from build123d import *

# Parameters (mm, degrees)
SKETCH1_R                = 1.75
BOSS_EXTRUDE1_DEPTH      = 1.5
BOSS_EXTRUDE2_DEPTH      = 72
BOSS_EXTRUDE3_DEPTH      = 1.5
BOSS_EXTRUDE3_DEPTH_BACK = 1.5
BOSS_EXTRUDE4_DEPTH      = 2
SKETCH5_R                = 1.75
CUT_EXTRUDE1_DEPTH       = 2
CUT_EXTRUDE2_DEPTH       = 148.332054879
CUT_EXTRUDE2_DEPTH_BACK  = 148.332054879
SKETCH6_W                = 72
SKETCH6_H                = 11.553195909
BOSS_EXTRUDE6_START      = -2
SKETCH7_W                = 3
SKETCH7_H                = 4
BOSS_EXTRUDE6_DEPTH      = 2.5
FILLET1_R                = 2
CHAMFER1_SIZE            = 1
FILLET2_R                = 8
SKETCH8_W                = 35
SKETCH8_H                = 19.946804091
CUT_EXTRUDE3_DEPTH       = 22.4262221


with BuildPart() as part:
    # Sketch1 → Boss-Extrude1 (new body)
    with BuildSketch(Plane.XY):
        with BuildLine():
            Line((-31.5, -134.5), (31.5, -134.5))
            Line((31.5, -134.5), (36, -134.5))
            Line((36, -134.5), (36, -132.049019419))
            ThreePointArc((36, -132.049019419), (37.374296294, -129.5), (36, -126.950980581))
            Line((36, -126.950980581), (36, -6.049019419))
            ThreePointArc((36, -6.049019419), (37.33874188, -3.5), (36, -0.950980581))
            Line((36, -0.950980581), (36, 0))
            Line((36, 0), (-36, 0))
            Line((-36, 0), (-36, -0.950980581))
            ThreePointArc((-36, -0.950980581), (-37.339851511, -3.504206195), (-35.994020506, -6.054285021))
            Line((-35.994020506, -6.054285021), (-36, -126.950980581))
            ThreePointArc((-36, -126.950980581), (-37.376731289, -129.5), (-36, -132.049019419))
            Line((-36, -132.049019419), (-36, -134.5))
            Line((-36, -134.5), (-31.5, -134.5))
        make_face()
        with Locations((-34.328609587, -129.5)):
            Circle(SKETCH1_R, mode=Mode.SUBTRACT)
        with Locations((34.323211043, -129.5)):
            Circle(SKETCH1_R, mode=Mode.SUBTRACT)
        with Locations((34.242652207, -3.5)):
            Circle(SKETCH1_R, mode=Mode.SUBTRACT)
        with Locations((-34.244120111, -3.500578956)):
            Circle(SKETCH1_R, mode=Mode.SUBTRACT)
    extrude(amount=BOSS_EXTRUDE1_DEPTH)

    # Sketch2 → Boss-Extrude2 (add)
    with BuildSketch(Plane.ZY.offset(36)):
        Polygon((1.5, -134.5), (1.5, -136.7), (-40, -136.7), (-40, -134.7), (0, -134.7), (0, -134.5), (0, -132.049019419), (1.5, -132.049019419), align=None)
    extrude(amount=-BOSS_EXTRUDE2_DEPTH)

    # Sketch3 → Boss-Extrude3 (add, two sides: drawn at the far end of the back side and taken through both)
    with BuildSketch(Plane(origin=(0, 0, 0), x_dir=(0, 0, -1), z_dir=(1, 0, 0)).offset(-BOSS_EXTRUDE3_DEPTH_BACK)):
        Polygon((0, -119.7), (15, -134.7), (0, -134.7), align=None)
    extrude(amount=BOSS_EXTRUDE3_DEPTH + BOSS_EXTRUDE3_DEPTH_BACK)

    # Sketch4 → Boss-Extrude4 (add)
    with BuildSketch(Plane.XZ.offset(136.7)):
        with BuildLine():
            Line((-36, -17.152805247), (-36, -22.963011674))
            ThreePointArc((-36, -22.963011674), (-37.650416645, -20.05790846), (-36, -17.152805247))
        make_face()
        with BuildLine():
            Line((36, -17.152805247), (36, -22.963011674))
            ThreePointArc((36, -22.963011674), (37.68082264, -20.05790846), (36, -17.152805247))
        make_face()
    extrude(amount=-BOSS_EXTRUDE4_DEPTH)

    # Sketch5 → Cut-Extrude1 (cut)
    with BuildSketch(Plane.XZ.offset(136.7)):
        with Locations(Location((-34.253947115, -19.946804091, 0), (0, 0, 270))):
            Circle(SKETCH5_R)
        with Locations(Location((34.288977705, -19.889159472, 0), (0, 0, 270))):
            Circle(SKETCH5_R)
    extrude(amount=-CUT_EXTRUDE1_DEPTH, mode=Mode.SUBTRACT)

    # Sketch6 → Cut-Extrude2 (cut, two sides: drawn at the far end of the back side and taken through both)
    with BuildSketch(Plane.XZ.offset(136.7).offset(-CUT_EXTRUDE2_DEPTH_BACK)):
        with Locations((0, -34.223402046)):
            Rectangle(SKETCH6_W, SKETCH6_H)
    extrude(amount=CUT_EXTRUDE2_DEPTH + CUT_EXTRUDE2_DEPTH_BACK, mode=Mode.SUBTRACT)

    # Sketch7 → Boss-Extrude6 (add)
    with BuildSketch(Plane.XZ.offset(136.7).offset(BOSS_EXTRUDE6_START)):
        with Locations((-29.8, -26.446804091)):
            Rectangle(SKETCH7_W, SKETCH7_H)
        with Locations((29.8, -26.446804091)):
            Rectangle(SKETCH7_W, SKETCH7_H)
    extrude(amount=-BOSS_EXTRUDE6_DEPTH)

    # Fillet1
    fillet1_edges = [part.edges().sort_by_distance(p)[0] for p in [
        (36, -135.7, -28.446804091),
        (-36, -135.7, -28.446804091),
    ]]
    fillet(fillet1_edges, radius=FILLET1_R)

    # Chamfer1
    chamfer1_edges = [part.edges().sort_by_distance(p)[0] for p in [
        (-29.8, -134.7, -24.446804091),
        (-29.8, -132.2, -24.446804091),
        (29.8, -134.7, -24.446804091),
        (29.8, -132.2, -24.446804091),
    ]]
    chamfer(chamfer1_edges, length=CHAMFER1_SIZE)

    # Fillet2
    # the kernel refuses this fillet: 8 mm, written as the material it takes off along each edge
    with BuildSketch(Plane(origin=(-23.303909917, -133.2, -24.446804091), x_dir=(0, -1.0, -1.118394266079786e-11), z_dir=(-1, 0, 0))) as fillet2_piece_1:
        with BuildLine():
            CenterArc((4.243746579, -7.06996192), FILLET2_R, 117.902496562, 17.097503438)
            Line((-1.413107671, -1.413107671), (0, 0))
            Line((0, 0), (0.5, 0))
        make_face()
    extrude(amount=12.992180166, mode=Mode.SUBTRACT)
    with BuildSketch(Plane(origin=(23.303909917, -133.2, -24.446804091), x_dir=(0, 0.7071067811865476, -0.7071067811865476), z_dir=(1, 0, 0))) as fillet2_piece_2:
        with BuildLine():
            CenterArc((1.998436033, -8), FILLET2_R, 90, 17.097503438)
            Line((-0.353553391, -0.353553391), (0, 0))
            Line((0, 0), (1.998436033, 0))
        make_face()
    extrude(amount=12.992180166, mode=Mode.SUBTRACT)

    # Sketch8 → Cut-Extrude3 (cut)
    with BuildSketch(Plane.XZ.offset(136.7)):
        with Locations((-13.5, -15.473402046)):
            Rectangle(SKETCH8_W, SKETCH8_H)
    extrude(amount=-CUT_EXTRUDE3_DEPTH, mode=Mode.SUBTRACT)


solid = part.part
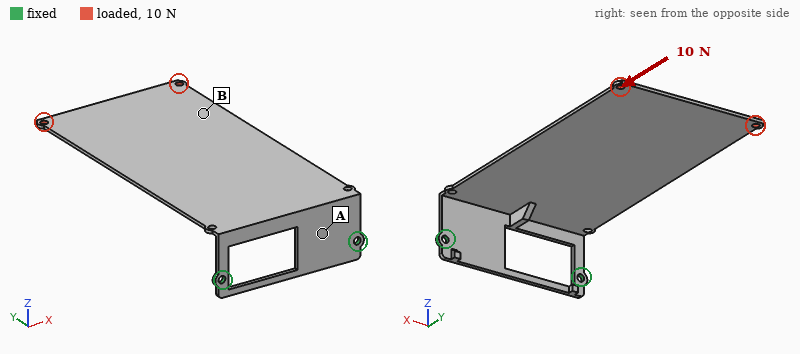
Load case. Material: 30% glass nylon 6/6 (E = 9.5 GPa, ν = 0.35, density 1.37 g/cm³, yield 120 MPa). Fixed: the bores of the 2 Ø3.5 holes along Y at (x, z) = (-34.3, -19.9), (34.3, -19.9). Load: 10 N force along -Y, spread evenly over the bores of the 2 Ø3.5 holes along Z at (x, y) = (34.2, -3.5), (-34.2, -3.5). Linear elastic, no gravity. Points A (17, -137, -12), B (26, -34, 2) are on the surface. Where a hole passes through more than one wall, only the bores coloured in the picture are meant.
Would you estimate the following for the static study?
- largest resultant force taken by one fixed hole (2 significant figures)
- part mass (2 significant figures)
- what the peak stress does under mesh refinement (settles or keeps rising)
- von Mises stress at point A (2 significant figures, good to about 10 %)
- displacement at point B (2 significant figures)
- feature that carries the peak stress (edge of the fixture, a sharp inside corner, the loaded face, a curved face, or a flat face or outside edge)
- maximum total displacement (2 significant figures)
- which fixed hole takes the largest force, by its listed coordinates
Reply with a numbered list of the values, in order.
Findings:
1. 5.4 N
2. 24 g
3. keeps rising
4. 2.7 MPa
5. 1.2 mm
6. edge of the fixture
7. 1.7 mm
8. (34.3, -19.9)
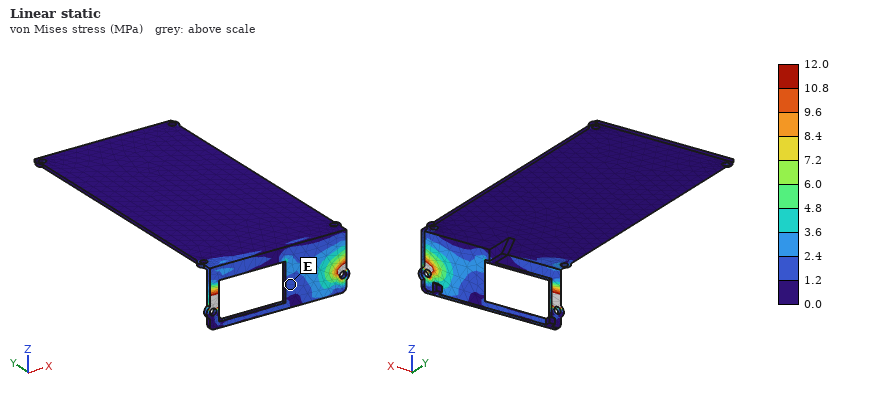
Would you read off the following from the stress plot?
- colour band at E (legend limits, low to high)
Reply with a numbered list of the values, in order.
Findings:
1. 1.2 to 2.4 MPa
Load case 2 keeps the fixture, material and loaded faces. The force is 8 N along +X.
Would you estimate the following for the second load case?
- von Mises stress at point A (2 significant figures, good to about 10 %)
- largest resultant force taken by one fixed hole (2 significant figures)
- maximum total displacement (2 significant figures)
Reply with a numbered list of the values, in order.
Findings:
1. 4.7 MPa
2. 17 N
3. 1.9 mm
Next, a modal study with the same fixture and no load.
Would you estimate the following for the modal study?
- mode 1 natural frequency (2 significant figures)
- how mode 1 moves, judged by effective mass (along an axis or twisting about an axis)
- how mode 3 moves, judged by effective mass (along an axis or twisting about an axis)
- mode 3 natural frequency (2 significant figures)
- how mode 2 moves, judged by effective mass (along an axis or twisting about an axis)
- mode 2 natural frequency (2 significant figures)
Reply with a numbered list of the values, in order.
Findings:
1. 29 Hz
2. along Z
3. along X
4. 150 Hz
5. along X
6. 120 Hz
